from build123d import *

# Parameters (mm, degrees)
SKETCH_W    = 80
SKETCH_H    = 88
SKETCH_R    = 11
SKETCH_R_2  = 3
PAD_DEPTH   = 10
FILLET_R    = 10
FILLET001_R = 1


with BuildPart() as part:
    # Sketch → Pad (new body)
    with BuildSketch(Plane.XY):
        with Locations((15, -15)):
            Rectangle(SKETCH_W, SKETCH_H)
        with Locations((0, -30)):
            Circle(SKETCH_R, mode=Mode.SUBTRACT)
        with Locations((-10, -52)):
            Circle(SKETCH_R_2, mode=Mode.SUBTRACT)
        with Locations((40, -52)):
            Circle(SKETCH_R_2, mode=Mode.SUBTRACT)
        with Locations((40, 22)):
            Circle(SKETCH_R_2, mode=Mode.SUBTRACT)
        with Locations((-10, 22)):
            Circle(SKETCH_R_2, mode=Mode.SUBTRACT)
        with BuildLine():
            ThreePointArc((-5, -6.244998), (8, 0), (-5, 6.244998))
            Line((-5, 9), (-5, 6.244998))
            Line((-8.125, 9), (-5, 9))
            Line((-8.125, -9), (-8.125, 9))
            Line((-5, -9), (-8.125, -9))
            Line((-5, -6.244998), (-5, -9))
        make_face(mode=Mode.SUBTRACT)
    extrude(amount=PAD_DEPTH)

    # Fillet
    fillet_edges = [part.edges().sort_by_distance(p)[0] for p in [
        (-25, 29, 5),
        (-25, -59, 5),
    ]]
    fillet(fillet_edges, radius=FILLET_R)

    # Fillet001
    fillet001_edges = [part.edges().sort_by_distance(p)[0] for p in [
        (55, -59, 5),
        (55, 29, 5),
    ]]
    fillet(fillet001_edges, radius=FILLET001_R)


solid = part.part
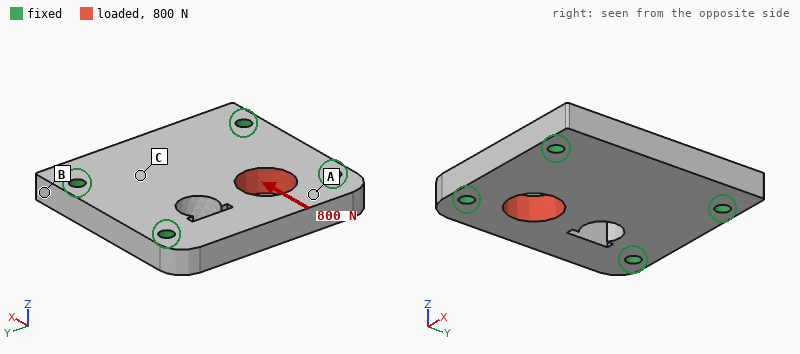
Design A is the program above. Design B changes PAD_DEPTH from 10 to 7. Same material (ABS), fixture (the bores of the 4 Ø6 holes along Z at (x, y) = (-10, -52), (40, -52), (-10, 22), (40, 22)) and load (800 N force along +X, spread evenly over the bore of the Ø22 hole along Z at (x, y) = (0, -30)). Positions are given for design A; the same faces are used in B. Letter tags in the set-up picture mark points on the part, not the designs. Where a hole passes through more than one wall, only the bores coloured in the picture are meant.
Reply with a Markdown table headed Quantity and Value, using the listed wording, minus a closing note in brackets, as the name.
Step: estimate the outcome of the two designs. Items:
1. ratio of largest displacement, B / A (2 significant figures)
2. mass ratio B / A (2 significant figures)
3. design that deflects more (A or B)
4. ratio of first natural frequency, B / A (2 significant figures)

| Quantity | Value |
|---|---|
| ratio of largest displacement, B / A | 1.4 |
| mass ratio B / A | 0.70 |
| design that deflects more | B |
| ratio of first natural frequency, B / A | 0.77 |
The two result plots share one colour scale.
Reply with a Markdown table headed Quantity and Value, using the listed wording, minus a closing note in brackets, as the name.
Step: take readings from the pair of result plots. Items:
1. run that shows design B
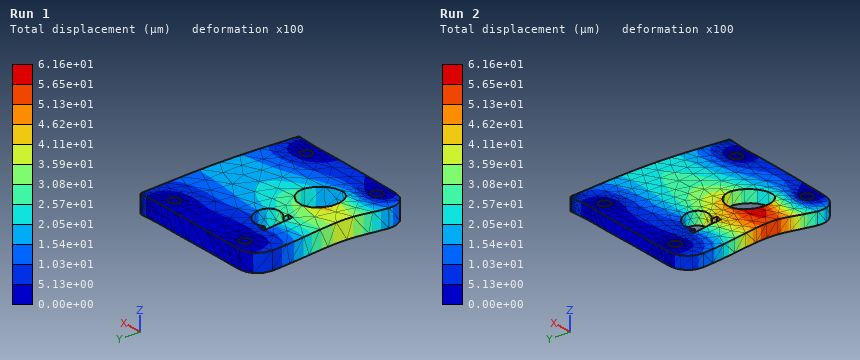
| Quantity | Value |
|---|---|
| run that shows design B | Run 2 |
